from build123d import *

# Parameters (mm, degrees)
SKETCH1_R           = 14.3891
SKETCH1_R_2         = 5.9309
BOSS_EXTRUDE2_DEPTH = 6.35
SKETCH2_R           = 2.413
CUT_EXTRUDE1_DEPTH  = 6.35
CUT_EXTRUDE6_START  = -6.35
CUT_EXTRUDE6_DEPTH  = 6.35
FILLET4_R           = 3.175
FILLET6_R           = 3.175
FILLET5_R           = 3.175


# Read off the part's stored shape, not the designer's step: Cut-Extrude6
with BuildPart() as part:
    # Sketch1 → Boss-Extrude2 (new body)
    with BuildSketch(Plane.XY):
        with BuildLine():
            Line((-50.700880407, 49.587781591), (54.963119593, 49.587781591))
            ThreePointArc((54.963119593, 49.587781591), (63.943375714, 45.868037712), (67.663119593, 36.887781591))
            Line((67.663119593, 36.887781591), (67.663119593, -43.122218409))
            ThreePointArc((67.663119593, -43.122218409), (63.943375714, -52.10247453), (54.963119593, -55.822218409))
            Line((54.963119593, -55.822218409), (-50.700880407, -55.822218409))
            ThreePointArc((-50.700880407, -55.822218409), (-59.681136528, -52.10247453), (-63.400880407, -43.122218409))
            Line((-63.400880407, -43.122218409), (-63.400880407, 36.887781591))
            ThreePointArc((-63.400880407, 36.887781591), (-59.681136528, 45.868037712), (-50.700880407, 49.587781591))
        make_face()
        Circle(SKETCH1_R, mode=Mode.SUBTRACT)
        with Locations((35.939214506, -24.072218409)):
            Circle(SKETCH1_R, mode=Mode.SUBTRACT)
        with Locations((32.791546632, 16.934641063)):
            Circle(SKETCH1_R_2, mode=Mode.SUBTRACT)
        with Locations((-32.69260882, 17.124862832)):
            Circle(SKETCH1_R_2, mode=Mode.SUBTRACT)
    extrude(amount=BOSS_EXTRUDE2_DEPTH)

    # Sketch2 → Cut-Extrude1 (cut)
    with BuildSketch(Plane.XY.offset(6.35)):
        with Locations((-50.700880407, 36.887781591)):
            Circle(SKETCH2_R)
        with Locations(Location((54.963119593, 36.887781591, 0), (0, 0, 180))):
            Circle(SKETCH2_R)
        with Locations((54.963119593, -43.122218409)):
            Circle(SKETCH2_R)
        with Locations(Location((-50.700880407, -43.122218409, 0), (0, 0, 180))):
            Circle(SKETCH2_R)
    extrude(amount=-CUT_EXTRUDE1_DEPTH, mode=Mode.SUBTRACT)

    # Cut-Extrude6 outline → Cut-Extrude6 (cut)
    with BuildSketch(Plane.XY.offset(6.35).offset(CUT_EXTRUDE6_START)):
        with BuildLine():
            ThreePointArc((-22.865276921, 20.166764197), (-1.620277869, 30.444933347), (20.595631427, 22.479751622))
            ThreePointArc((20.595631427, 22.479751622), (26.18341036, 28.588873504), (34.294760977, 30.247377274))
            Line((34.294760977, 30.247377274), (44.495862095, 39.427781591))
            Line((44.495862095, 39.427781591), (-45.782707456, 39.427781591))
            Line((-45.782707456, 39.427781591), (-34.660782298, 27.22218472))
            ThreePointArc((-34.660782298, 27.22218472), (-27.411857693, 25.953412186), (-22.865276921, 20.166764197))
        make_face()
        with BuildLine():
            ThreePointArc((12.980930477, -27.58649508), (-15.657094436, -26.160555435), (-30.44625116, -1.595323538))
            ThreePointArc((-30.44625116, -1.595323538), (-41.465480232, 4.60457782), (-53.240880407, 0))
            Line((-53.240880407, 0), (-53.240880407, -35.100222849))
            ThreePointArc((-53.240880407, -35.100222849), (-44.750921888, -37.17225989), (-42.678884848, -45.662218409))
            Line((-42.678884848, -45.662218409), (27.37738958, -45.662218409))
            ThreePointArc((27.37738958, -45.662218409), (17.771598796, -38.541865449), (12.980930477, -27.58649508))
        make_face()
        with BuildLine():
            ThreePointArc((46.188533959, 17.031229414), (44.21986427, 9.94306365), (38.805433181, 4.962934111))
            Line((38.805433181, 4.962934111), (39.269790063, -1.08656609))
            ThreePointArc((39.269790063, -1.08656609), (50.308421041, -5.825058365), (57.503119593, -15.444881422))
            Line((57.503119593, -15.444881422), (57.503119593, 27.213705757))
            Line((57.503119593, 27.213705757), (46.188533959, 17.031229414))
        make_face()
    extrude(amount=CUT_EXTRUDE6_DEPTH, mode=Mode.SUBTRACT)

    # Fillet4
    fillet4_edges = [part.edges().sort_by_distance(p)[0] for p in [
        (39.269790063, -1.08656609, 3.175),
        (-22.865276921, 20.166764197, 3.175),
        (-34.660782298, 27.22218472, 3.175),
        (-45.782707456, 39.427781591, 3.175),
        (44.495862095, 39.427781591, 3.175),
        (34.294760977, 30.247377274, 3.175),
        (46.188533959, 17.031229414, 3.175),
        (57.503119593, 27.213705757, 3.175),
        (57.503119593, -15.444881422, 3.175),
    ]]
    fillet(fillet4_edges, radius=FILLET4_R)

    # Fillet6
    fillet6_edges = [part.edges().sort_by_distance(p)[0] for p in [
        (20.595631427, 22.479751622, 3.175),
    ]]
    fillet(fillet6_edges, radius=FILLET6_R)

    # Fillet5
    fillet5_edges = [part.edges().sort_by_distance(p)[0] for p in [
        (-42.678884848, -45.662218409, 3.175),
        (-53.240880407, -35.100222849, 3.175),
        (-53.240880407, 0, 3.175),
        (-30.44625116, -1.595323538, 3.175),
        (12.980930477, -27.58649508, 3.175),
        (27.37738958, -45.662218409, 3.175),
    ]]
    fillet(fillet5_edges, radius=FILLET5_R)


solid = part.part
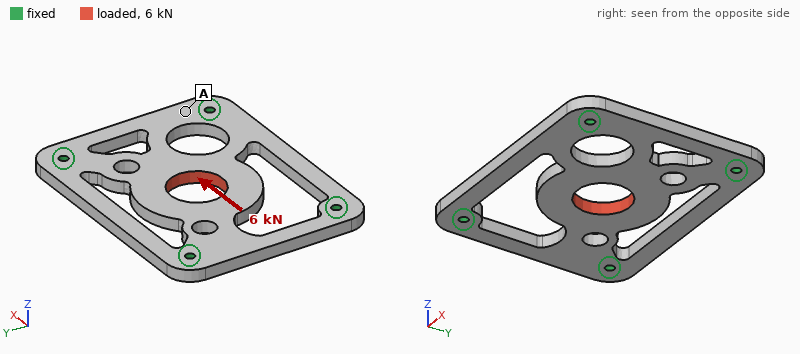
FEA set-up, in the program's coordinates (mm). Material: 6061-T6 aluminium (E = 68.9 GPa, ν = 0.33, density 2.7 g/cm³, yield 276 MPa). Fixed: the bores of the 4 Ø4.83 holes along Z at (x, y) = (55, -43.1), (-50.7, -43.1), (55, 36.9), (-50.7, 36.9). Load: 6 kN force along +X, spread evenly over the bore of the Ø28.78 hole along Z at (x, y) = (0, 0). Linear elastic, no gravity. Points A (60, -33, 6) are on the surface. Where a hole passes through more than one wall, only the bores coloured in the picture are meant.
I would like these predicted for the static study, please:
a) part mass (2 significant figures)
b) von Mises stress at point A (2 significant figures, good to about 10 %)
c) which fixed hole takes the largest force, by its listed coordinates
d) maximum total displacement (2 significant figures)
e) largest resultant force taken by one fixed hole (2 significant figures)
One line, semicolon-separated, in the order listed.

150 g; 10 MPa; (55, 36.9); 39 µm; 2.8 kN
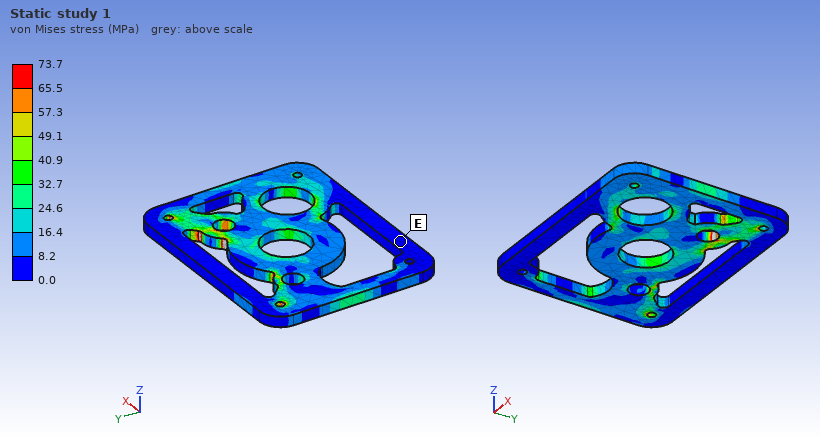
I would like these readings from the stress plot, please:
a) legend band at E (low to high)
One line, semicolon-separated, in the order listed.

0.0 to 8.2 MPa
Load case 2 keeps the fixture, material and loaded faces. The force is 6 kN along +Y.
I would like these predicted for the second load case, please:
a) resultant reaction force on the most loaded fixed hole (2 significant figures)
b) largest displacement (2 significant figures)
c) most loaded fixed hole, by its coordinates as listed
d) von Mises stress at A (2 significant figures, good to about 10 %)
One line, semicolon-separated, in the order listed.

3.2 kN; 54 µm; (55, 36.9); 12 MPa
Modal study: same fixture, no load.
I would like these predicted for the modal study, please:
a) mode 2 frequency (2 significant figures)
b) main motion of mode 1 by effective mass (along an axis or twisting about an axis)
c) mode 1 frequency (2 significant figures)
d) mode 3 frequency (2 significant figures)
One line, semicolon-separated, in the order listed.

3100 Hz; along Z; 1900 Hz; 3300 Hz
